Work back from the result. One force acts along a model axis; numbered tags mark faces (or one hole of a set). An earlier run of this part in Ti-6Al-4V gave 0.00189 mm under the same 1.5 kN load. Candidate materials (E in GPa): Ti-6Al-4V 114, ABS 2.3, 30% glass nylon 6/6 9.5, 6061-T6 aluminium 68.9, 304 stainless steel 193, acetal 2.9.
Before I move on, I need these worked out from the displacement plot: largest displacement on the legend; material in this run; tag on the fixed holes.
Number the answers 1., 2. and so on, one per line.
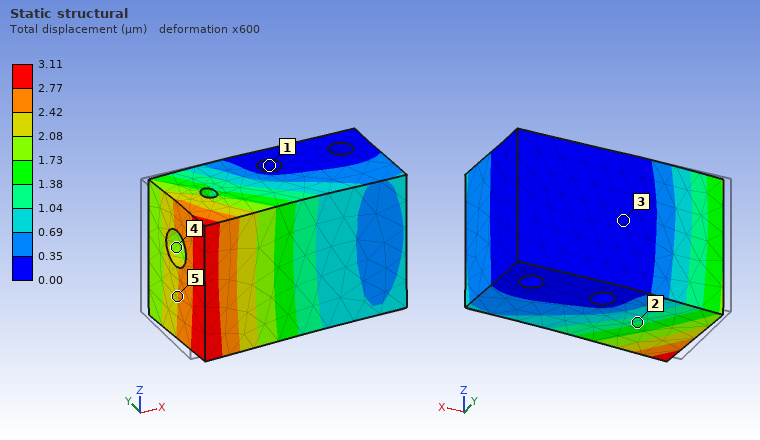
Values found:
1. 3.11 µm
2. 6061-T6 aluminium
3. 1
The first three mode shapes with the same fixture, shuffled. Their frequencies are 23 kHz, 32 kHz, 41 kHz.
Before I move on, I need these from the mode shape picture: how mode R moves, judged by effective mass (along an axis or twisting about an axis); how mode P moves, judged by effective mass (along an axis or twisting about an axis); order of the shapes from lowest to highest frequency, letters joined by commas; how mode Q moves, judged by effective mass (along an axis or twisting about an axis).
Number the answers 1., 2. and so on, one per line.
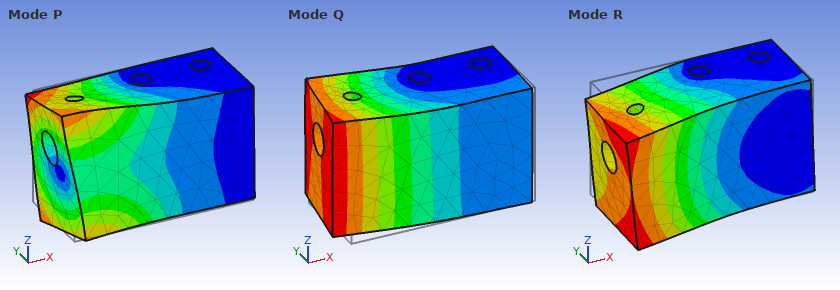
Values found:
1. along Z
2. twisting about X
3. Q, R, P
4. along Y
